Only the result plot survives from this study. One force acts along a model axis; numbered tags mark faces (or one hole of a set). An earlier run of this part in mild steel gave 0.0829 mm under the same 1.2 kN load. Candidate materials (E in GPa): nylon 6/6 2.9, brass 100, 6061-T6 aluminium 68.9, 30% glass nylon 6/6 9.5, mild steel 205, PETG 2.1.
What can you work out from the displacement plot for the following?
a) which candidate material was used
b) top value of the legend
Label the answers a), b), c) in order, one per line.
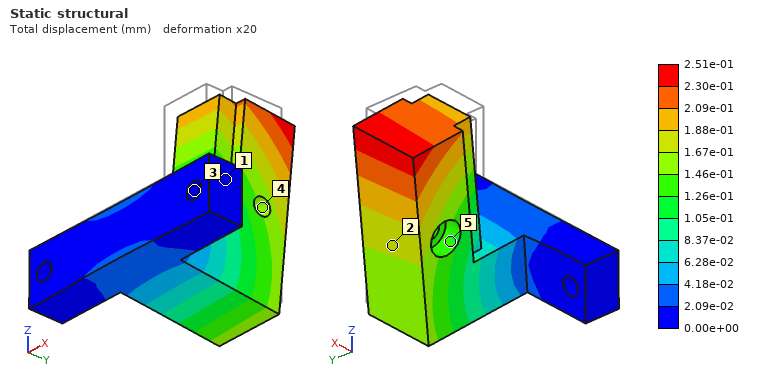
a) 6061-T6 aluminium
b) 2.51e-01 mm
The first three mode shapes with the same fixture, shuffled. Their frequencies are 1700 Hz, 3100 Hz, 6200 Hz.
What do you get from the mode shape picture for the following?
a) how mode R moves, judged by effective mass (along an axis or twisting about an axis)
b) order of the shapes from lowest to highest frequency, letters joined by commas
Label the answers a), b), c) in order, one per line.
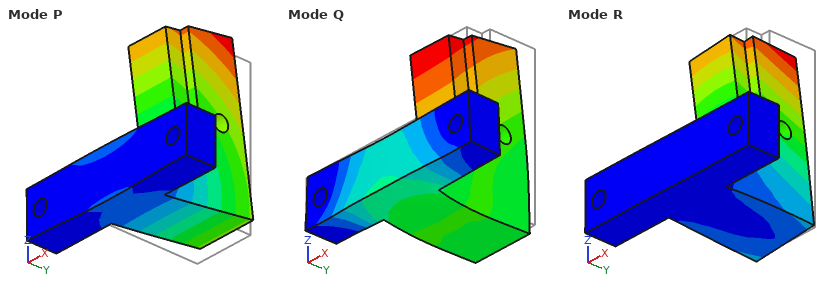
a) along X
b) P, R, Q
